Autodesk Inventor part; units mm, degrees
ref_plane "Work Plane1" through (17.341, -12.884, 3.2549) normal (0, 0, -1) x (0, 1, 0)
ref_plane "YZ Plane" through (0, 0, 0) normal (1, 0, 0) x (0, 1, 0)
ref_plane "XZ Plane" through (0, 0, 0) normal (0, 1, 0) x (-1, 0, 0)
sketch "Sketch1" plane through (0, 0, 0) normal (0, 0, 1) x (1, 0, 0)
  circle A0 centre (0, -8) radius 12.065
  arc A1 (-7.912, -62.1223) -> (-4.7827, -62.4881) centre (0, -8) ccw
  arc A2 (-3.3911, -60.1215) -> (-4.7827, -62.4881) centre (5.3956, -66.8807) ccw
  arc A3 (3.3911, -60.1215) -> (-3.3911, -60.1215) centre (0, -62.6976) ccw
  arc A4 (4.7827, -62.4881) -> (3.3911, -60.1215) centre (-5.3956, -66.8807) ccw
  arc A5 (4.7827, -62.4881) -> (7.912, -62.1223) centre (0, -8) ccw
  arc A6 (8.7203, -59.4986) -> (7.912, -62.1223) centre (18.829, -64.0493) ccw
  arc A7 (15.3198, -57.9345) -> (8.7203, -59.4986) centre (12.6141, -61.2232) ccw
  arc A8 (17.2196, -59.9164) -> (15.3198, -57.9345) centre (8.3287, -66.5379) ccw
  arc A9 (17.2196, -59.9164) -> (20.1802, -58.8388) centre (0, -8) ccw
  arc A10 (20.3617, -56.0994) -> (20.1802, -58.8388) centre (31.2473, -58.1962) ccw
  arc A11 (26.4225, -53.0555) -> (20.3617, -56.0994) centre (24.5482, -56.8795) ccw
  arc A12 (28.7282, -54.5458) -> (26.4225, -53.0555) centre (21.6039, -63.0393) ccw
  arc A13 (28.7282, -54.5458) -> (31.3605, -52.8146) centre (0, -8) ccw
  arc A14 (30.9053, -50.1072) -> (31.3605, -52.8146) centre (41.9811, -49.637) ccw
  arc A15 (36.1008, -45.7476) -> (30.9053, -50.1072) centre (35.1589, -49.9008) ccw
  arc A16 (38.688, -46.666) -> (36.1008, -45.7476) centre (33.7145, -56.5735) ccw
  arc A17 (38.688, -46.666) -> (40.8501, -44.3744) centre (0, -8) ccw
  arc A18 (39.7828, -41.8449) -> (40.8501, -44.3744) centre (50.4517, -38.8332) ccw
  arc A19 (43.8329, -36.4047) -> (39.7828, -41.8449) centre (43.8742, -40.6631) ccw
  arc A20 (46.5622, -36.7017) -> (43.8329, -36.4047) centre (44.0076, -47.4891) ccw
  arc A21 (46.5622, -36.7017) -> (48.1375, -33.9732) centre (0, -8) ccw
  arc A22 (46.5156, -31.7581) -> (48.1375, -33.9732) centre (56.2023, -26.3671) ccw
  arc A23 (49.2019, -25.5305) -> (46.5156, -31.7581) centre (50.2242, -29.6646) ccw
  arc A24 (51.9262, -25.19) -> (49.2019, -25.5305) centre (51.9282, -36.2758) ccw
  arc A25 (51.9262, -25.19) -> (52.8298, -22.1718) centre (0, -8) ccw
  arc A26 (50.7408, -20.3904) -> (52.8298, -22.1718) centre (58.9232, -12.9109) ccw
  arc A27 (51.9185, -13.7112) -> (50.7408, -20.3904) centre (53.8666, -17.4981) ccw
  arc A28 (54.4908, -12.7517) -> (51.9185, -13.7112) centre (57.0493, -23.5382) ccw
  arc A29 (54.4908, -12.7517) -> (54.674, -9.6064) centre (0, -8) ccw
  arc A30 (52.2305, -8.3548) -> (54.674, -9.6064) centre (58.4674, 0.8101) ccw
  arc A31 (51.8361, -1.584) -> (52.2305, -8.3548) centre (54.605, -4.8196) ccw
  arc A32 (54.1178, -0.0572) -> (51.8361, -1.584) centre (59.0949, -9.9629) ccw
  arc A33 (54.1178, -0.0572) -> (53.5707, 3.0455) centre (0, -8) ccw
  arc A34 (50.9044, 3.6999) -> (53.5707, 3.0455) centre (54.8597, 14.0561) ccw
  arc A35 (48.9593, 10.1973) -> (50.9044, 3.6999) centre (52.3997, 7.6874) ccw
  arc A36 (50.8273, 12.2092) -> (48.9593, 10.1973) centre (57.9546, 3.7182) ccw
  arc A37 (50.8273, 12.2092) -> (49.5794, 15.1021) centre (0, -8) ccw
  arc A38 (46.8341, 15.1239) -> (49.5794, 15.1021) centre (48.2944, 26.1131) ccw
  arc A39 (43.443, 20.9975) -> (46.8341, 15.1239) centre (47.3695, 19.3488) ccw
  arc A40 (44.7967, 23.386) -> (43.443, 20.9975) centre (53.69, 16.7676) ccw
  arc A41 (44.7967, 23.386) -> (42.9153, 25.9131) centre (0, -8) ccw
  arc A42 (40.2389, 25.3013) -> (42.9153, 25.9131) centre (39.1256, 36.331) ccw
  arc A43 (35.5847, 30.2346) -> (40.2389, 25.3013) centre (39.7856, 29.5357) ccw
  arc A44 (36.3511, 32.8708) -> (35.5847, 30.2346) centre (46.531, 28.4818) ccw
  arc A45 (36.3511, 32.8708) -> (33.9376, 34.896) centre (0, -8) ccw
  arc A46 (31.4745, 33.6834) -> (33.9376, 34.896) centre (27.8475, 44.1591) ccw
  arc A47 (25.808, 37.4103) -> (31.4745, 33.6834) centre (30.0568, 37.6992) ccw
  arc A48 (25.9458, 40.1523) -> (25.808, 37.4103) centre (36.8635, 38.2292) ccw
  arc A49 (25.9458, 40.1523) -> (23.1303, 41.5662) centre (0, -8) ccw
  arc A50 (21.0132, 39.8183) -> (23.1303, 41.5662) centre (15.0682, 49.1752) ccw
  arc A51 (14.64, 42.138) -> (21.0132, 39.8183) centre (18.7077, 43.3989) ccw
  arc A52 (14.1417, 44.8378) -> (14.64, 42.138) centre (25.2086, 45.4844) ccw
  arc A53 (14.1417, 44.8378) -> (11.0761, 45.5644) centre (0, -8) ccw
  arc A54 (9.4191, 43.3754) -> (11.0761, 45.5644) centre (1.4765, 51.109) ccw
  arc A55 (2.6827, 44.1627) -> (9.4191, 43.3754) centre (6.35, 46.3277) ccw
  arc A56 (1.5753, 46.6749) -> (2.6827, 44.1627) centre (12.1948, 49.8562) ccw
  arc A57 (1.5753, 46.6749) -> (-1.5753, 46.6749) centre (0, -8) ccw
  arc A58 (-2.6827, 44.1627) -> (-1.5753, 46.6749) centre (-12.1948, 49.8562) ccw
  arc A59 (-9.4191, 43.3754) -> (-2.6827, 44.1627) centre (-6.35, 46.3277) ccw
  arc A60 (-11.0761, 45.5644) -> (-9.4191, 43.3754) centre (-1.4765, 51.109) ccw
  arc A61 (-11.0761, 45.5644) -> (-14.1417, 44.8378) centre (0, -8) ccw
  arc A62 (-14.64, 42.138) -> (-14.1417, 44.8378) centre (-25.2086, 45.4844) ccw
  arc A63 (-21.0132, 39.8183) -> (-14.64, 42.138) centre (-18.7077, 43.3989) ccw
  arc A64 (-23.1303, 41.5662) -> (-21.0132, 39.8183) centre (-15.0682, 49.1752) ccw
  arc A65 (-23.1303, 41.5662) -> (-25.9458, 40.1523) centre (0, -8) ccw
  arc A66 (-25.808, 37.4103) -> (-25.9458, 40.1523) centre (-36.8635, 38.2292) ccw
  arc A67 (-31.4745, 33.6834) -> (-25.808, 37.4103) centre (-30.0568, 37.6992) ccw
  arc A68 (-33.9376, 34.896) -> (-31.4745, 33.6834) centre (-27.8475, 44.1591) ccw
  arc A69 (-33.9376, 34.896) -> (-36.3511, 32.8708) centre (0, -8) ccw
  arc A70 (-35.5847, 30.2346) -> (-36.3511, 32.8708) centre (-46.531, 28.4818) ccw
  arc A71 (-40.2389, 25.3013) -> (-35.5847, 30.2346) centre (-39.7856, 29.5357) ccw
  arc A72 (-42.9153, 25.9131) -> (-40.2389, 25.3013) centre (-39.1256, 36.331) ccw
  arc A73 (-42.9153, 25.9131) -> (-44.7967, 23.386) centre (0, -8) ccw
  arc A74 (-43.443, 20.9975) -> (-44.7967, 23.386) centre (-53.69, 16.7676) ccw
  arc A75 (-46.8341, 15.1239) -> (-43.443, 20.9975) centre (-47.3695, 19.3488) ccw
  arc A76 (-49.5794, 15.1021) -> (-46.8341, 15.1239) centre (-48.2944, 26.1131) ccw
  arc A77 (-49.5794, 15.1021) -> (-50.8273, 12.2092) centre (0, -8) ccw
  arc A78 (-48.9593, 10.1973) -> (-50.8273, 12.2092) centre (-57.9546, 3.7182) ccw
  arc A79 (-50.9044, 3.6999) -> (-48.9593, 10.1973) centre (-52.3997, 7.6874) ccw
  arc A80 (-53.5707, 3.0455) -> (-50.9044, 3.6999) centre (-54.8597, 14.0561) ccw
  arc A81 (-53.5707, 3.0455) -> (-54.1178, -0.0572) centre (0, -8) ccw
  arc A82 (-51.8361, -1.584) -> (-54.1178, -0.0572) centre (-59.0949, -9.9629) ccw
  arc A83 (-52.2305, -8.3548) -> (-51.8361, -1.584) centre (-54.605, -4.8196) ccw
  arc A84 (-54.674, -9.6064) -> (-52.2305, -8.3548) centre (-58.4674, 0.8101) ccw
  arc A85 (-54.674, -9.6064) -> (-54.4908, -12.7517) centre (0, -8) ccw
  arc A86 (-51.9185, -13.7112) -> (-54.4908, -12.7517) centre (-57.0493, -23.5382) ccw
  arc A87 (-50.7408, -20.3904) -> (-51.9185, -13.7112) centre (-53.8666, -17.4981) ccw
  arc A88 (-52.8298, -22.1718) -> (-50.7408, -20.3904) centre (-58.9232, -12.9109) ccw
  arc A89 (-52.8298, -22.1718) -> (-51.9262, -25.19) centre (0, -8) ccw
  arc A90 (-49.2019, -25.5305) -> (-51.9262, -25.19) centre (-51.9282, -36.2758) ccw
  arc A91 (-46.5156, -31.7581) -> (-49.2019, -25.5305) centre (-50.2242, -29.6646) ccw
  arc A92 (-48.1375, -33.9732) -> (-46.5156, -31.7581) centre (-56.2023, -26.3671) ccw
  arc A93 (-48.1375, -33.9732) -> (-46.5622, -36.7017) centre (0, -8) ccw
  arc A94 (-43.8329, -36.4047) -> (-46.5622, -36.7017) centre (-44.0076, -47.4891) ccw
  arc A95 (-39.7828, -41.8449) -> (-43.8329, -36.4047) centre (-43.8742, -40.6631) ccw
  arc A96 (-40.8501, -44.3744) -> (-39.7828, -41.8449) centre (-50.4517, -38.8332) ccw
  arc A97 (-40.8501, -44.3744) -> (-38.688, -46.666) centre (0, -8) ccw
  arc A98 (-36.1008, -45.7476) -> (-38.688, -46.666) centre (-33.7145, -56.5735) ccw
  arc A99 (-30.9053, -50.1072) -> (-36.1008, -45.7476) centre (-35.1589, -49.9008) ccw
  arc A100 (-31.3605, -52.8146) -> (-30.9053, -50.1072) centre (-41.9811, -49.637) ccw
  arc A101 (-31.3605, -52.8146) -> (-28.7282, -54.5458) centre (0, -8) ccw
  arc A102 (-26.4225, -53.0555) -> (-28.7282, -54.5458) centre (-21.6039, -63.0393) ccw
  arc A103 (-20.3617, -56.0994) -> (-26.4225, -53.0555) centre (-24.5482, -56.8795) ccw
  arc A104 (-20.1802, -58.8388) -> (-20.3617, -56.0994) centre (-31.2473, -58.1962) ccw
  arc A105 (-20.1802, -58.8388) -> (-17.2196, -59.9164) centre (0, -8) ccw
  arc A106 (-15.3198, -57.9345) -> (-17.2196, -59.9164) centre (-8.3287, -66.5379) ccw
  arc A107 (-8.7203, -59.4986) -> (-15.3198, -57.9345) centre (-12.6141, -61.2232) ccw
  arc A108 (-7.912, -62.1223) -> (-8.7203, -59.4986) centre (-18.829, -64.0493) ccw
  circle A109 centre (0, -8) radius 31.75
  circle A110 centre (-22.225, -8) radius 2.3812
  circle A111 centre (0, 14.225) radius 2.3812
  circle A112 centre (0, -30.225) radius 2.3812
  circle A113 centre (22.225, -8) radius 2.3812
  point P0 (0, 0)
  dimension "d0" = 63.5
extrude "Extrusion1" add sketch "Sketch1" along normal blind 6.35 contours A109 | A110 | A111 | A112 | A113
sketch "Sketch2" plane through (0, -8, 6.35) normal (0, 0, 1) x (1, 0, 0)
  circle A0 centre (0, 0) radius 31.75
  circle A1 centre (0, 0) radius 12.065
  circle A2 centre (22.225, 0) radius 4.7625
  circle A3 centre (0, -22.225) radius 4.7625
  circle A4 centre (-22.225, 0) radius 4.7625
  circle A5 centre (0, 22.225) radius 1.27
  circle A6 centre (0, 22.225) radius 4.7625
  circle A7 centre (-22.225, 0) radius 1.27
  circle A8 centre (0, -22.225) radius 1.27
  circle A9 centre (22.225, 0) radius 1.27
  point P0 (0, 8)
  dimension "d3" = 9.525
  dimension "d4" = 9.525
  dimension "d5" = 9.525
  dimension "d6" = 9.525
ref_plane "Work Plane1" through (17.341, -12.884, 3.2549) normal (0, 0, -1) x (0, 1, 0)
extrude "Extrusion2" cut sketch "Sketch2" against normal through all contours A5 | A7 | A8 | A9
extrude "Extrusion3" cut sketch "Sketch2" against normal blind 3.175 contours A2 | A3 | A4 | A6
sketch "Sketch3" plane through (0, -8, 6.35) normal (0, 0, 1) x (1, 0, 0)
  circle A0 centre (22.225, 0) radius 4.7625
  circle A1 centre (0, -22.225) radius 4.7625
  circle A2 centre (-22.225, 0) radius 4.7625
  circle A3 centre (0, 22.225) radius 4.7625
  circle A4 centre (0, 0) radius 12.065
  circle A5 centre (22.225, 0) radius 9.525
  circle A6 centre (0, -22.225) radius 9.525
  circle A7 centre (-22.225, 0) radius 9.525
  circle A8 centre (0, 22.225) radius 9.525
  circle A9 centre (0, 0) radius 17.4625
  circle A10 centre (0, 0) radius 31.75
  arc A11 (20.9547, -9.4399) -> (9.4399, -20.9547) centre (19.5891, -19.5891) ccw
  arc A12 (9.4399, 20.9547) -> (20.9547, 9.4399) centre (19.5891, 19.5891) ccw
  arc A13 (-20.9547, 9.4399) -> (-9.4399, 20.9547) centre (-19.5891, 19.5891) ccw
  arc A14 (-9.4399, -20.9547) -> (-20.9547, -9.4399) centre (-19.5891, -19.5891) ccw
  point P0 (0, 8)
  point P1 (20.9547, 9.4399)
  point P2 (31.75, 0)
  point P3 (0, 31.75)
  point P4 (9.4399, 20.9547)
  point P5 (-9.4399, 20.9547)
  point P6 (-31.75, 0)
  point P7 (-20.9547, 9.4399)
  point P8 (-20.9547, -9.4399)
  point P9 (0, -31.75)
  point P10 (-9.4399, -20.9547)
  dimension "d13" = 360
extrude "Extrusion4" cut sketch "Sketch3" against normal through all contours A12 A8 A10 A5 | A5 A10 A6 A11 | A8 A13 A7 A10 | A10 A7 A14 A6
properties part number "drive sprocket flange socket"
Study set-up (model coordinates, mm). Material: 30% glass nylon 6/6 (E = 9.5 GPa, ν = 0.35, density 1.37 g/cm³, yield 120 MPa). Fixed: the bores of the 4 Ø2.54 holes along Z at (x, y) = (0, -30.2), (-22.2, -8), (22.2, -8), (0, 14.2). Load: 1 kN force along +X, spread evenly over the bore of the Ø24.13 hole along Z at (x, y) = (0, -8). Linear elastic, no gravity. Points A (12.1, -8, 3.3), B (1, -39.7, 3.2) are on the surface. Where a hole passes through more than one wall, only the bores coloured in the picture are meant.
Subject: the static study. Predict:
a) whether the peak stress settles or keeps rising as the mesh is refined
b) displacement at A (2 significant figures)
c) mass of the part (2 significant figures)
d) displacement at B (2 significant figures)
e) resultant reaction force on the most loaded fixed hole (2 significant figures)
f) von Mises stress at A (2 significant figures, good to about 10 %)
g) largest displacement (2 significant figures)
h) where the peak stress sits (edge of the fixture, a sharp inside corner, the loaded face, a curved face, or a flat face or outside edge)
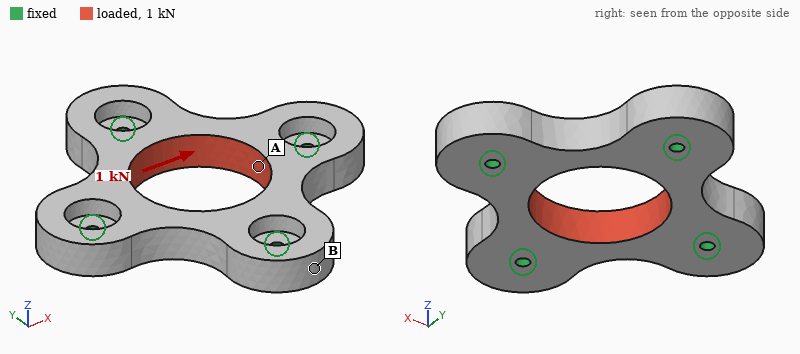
keeps rising
9.3 µm
12 g
7.3 µm
340 N
9.0 MPa
18 µm
edge of the fixture
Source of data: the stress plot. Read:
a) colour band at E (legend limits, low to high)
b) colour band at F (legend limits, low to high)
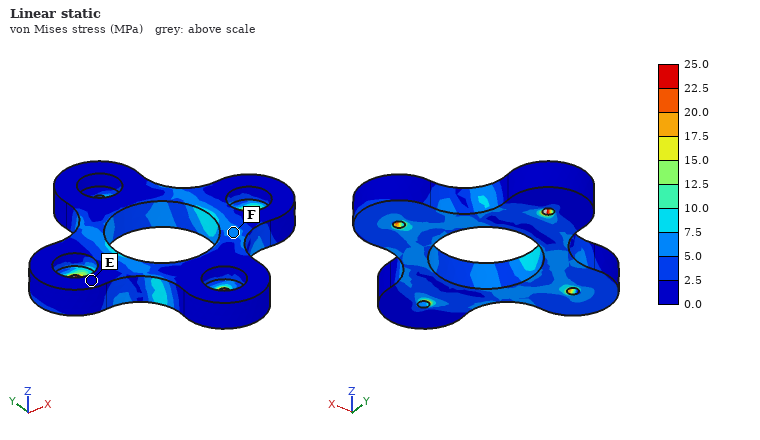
0.0 to 2.5 MPa
5.0 to 7.5 MPa
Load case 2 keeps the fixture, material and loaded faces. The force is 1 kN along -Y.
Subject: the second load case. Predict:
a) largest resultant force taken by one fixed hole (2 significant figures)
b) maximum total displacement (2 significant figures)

340 N
18 µm
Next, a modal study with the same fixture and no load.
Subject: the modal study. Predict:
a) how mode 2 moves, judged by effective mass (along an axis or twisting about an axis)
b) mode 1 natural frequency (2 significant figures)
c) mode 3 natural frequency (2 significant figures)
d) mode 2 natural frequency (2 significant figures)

along Z
8300 Hz
9700 Hz
9000 Hz
